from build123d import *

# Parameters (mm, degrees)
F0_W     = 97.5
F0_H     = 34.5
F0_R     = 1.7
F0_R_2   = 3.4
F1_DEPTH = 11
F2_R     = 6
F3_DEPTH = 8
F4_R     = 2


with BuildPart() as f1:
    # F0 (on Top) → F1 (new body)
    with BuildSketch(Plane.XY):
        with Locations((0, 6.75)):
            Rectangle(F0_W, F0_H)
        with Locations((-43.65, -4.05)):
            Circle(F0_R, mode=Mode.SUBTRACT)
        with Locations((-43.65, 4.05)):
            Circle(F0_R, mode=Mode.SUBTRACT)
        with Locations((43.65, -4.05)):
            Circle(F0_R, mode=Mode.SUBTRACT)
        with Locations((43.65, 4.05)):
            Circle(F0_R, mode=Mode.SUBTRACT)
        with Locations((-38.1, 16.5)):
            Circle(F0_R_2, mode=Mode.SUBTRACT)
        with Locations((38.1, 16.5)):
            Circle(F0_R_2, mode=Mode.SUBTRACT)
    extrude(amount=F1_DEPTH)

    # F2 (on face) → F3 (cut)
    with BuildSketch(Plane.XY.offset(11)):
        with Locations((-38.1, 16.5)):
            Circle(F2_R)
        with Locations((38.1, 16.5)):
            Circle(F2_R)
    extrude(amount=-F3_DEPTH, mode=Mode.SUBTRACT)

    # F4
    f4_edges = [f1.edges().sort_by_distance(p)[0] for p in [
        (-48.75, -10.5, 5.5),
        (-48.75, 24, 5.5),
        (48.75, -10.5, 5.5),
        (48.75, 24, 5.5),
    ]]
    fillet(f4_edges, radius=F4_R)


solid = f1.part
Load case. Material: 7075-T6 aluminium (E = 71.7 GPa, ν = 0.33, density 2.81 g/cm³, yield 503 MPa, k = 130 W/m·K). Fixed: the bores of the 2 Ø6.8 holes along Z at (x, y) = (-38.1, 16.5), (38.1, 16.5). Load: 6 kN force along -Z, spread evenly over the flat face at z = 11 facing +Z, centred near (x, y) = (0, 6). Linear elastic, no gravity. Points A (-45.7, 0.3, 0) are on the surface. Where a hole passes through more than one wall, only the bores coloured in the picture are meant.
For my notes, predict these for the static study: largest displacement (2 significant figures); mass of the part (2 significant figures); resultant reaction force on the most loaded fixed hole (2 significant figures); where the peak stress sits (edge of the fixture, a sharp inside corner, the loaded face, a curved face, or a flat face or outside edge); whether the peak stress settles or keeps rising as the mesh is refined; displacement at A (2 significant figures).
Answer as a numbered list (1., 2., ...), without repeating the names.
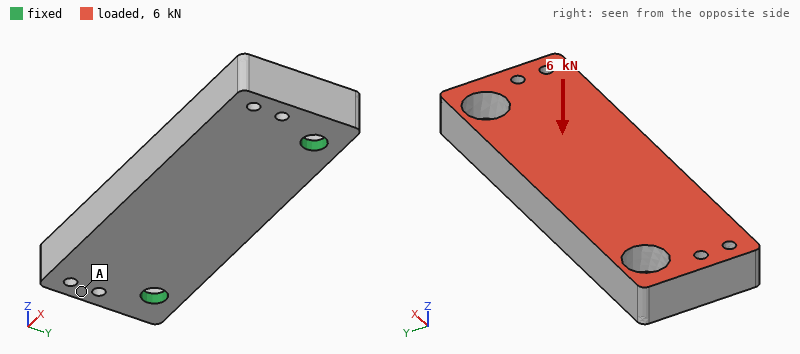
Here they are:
1. 0.26 mm
2. 97 g
3. 3.6 kN
4. edge of the fixture
5. keeps rising
6. 0.100 mm
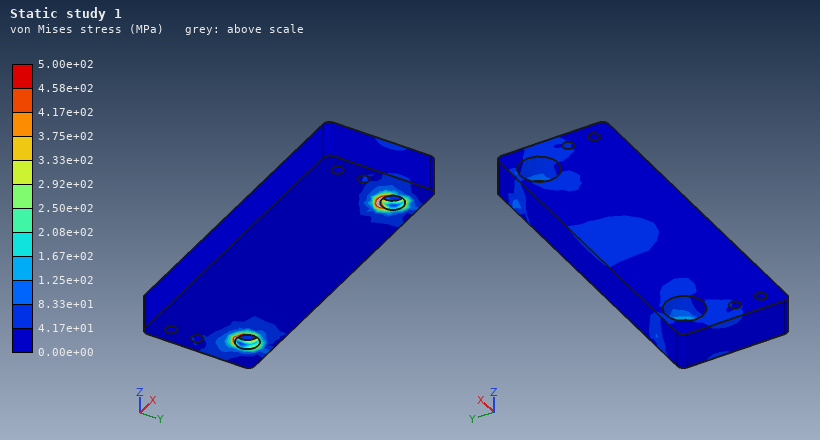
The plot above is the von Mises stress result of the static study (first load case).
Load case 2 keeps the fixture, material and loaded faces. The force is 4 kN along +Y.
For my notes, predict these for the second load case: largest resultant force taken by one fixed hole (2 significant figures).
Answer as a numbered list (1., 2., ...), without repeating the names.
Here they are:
1. 2.1 kN
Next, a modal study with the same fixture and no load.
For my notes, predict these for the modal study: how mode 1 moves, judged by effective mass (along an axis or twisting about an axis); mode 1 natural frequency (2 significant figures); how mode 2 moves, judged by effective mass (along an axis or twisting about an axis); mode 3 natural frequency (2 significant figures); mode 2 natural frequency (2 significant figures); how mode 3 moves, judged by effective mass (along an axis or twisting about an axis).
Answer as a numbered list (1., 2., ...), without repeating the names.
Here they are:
1. along Z
2. 3000 Hz
3. along Z
4. 7300 Hz
5. 6800 Hz
6. twisting about Y
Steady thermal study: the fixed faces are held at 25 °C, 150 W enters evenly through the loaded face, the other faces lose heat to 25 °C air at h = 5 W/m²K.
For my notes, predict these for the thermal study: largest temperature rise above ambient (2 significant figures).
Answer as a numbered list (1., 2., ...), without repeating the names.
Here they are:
1. 60 K
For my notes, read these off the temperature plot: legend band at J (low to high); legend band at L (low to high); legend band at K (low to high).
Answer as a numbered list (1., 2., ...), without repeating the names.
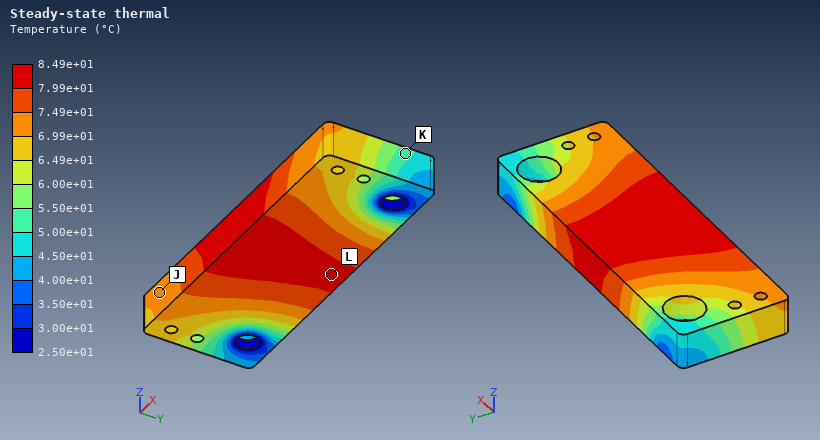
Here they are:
1. 6.99e+01 to 7.49e+01 °C
2. 7.99e+01 to 8.49e+01 °C
3. 5.00e+01 to 5.50e+01 °C
